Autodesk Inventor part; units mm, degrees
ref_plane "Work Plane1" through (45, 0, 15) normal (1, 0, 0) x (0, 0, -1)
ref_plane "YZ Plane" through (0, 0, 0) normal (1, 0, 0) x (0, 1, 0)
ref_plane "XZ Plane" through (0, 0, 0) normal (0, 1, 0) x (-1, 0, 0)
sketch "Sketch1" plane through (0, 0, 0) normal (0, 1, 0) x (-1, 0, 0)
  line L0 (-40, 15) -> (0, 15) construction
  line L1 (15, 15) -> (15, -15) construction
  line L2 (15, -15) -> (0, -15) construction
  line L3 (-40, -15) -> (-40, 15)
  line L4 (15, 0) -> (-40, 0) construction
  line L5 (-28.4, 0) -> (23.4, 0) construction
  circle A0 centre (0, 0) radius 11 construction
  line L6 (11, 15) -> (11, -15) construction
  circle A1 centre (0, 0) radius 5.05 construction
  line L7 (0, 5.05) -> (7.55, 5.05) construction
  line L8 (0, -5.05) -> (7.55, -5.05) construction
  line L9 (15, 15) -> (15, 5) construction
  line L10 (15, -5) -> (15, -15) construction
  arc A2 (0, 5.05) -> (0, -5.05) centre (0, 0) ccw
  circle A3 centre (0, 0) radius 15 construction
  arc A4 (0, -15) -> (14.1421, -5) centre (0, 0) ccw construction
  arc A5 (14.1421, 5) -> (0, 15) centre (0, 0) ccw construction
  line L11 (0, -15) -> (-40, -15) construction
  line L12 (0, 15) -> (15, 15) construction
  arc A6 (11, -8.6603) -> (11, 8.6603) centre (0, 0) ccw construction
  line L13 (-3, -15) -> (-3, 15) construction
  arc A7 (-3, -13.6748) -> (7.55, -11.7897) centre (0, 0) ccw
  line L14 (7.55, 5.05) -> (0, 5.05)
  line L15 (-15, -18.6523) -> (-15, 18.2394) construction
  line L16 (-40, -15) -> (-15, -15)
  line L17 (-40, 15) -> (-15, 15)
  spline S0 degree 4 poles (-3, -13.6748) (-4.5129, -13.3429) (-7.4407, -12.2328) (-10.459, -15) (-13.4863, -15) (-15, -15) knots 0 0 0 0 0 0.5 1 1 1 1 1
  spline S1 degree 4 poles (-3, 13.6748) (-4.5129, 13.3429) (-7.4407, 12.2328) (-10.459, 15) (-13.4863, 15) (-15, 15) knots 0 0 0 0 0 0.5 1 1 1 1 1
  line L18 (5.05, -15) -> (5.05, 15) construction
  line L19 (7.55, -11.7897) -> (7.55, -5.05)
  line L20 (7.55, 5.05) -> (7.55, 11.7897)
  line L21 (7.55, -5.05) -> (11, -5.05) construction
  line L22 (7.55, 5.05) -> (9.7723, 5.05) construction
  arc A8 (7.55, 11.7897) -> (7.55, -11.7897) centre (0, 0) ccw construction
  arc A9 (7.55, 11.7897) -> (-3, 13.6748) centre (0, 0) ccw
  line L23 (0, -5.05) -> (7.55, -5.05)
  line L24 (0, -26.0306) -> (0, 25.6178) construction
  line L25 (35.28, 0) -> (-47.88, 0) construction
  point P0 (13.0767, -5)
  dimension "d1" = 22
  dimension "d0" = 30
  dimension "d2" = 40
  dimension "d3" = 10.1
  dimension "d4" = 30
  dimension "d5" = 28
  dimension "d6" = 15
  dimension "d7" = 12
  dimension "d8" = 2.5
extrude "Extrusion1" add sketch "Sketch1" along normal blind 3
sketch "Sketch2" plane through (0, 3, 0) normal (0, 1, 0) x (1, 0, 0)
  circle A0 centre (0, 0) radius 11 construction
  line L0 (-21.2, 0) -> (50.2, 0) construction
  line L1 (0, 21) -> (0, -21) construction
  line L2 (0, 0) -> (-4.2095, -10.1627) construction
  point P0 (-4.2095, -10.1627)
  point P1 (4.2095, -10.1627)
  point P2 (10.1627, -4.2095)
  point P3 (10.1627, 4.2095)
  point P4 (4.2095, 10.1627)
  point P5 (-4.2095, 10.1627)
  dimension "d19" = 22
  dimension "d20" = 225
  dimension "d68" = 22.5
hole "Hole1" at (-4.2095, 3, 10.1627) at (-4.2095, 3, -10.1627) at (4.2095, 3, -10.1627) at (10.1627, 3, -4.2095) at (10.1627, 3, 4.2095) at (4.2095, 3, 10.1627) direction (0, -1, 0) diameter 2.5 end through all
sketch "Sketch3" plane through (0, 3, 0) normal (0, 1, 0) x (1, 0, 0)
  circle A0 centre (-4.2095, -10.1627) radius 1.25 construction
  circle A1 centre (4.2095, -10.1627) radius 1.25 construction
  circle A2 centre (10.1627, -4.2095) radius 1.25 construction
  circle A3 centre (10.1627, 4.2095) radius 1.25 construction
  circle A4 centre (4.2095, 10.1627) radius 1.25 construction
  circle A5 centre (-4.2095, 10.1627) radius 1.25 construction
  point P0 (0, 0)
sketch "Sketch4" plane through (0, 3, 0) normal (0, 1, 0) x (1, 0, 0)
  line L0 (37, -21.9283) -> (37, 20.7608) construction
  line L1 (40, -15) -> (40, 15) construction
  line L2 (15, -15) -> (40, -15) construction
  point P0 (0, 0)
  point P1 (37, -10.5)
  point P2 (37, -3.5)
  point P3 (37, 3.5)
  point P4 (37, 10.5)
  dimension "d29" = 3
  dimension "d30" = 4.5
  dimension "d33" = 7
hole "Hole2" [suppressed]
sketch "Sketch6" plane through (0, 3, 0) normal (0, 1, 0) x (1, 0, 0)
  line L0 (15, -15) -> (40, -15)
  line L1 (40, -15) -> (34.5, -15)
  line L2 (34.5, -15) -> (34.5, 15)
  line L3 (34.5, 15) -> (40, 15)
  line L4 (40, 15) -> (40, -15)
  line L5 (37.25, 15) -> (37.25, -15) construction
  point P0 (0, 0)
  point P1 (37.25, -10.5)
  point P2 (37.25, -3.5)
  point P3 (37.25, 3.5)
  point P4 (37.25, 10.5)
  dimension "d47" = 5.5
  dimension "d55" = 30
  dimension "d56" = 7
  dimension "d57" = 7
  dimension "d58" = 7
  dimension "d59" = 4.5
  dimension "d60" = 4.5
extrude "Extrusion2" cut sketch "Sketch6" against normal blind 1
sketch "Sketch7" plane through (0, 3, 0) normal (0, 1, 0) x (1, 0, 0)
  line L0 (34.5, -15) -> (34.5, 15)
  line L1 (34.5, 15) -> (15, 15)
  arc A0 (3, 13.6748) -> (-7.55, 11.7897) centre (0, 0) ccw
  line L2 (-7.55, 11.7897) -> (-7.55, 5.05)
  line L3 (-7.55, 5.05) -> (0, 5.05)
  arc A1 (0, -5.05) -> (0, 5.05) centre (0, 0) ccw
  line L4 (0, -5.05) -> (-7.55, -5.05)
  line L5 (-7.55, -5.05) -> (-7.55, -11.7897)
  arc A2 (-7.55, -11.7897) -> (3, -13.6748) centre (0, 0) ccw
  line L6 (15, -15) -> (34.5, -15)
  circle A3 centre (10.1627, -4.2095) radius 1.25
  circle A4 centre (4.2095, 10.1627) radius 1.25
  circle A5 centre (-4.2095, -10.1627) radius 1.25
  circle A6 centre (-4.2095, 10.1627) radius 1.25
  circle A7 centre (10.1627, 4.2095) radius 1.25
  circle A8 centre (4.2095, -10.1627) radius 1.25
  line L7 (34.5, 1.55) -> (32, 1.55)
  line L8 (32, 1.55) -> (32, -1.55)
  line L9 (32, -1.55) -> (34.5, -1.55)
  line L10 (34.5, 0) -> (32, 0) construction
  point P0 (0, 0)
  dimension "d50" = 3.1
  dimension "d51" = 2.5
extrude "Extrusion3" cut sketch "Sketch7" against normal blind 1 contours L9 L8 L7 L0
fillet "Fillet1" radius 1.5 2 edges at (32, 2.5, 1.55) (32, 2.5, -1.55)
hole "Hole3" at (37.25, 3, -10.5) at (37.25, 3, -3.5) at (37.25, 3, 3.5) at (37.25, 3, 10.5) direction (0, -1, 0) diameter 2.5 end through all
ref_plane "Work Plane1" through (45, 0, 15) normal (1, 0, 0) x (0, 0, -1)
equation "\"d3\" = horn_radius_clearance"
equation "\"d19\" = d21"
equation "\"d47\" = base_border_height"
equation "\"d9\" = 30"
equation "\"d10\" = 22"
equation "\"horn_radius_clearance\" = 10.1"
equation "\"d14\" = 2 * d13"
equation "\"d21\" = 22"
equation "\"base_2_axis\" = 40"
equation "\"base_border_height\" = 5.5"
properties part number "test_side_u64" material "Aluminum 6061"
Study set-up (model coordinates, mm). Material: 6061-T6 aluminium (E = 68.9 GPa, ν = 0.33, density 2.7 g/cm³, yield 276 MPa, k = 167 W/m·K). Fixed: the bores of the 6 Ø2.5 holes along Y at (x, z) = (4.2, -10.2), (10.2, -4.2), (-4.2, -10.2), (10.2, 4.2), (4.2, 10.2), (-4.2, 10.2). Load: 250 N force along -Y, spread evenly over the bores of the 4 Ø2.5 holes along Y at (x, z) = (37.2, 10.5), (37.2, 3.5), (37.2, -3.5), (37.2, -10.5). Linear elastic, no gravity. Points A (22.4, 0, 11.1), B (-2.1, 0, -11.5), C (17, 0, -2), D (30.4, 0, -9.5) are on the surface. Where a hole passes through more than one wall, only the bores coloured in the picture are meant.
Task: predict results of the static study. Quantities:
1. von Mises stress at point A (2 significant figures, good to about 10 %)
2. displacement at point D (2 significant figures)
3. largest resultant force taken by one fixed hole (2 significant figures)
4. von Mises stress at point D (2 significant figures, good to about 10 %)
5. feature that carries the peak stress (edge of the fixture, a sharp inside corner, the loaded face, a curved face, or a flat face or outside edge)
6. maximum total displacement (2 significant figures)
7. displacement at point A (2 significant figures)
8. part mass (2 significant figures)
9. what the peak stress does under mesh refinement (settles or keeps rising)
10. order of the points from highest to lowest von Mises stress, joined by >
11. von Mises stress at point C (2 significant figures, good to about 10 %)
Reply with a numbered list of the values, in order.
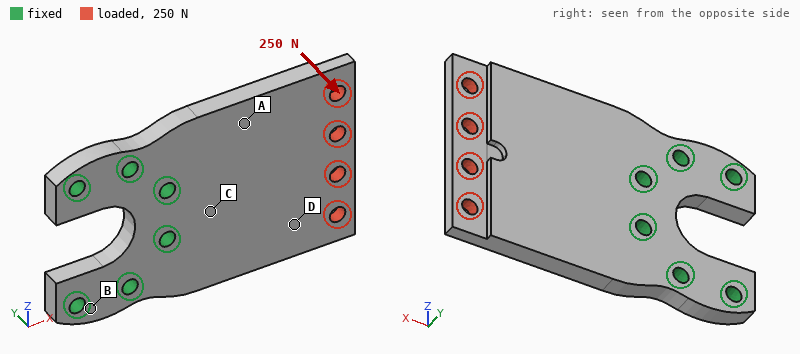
1. 80 MPa
2. 0.23 mm
3. 300 N
4. 40 MPa
5. edge of the fixture
6. 0.42 mm
7. 0.097 mm
8. 9.3 g
9. keeps rising
10. C > A > D > B
11. 110 MPa
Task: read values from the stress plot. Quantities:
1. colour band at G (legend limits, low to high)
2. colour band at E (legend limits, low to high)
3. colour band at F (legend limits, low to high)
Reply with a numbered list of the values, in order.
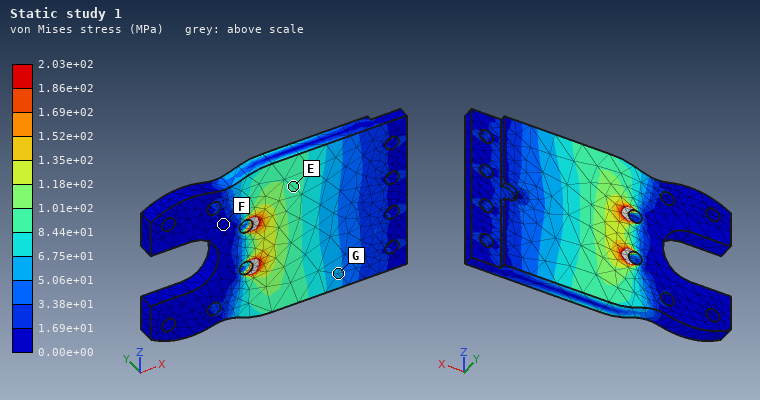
1. 5.06e+01 to 6.75e+01 MPa
2. 8.44e+01 to 1.01e+02 MPa
3. 0.00e+00 to 1.69e+01 MPa
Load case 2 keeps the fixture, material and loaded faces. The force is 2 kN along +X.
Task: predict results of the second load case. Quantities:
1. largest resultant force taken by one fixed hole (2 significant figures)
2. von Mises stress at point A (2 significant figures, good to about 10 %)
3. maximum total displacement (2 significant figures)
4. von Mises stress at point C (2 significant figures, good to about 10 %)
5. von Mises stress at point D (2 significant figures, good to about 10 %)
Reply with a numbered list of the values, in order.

1. 640 N
2. 42 MPa
3. 94 µm
4. 47 MPa
5. 44 MPa
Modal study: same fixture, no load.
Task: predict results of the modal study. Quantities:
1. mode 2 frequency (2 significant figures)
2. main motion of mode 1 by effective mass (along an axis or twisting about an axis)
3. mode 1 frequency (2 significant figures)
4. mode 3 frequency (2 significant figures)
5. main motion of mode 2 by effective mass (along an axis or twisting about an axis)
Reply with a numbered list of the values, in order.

1. 6100 Hz
2. along Y
3. 3100 Hz
4. 15 kHz
5. twisting about X
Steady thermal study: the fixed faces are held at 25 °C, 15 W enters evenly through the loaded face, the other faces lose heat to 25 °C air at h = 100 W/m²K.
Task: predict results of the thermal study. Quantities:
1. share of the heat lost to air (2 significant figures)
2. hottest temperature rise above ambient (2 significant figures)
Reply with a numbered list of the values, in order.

1. 19 %
2. 29 K
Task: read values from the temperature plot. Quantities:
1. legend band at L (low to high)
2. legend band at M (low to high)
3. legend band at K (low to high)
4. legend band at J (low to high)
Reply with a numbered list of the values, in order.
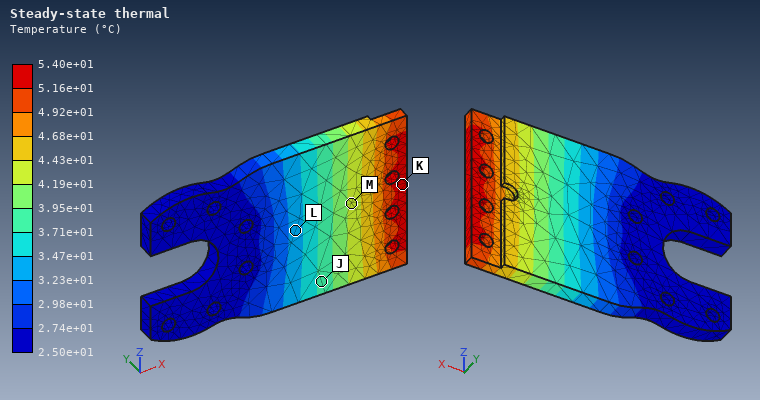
1. 3.23e+01 to 3.47e+01 °C
2. 4.19e+01 to 4.43e+01 °C
3. 5.16e+01 to 5.40e+01 °C
4. 3.71e+01 to 3.95e+01 °C
